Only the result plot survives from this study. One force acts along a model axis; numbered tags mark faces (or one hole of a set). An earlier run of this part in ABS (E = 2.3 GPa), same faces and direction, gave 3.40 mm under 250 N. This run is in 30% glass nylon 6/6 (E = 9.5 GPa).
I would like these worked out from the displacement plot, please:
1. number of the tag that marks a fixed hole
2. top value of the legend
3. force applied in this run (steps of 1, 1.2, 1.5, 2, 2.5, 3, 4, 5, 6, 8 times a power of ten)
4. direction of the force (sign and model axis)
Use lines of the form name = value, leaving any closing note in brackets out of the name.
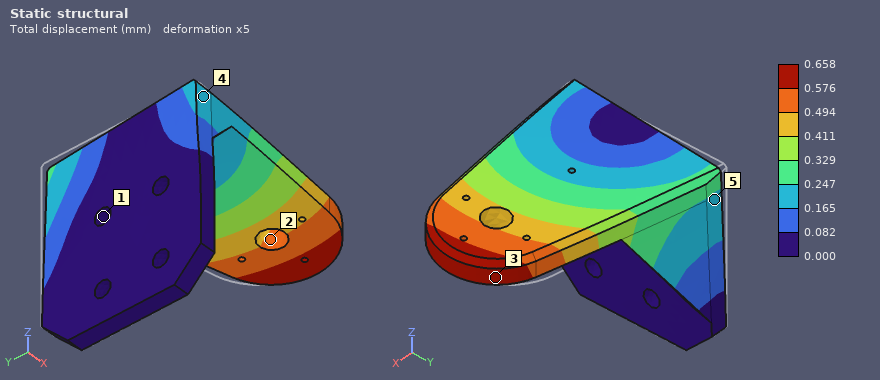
number of the tag that marks a fixed hole = 1
top value of the legend = 0.658 mm
force applied in this run = 200 N
direction of the force = -Y
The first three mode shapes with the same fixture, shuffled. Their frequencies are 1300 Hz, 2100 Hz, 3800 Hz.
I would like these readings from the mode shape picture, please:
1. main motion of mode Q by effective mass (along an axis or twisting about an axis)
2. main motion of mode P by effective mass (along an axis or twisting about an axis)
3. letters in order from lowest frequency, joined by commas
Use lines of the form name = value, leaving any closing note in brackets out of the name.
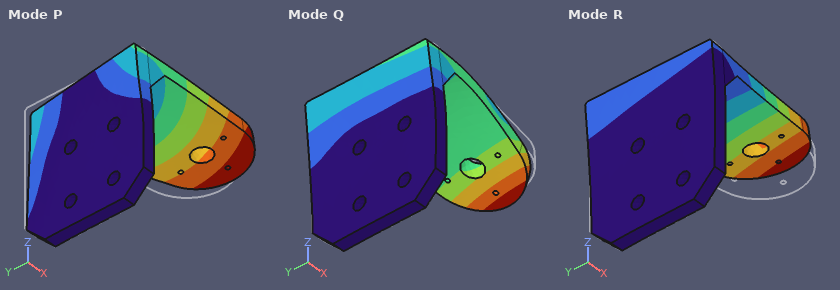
main motion of mode Q by effective mass = along X
main motion of mode P by effective mass = along Y
letters in order from lowest frequency, joined by commas = R, P, Q
